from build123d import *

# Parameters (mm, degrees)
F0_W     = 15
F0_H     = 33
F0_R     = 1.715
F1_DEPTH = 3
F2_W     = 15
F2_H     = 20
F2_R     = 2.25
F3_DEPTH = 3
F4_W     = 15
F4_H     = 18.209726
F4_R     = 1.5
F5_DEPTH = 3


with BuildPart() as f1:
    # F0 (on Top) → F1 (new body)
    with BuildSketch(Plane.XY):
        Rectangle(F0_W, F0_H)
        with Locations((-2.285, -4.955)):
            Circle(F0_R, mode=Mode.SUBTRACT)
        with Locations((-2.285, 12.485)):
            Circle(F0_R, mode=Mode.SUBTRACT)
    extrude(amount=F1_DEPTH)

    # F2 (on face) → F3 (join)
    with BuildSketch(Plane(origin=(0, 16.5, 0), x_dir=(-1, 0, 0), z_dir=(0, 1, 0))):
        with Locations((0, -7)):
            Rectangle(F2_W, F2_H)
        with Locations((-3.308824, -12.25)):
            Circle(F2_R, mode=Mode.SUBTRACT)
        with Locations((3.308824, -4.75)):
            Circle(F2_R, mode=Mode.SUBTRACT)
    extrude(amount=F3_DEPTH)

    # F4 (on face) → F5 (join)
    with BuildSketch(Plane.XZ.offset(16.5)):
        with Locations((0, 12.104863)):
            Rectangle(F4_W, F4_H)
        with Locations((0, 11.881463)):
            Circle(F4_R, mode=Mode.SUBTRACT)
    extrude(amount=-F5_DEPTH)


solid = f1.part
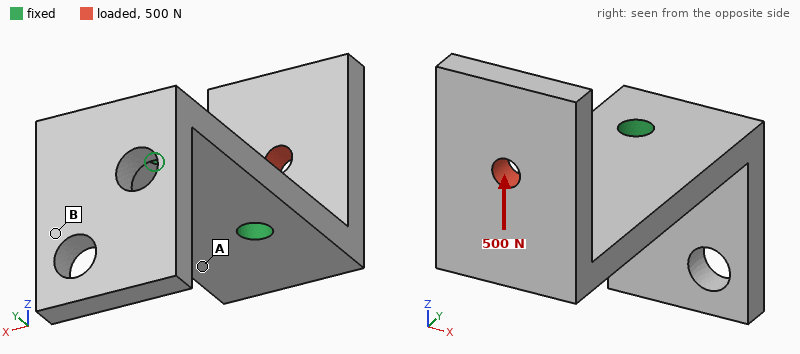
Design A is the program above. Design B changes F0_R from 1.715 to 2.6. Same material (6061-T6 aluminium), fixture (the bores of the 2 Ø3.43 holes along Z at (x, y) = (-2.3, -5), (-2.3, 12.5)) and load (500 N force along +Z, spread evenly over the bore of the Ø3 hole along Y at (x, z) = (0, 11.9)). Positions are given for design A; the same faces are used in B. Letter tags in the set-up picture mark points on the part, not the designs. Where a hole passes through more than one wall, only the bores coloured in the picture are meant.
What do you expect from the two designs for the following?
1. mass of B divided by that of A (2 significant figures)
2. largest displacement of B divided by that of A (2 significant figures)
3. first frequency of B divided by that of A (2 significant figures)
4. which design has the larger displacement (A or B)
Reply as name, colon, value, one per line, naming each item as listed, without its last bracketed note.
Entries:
mass of B divided by that of A: 0.98
largest displacement of B divided by that of A: 0.78
first frequency of B divided by that of A: 1.1
which design has the larger displacement: A
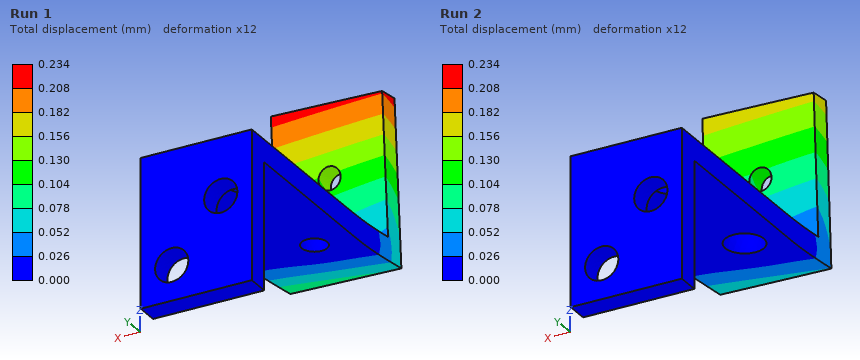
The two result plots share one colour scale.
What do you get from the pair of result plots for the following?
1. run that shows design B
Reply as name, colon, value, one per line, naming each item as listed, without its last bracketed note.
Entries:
run that shows design B: Run 2
